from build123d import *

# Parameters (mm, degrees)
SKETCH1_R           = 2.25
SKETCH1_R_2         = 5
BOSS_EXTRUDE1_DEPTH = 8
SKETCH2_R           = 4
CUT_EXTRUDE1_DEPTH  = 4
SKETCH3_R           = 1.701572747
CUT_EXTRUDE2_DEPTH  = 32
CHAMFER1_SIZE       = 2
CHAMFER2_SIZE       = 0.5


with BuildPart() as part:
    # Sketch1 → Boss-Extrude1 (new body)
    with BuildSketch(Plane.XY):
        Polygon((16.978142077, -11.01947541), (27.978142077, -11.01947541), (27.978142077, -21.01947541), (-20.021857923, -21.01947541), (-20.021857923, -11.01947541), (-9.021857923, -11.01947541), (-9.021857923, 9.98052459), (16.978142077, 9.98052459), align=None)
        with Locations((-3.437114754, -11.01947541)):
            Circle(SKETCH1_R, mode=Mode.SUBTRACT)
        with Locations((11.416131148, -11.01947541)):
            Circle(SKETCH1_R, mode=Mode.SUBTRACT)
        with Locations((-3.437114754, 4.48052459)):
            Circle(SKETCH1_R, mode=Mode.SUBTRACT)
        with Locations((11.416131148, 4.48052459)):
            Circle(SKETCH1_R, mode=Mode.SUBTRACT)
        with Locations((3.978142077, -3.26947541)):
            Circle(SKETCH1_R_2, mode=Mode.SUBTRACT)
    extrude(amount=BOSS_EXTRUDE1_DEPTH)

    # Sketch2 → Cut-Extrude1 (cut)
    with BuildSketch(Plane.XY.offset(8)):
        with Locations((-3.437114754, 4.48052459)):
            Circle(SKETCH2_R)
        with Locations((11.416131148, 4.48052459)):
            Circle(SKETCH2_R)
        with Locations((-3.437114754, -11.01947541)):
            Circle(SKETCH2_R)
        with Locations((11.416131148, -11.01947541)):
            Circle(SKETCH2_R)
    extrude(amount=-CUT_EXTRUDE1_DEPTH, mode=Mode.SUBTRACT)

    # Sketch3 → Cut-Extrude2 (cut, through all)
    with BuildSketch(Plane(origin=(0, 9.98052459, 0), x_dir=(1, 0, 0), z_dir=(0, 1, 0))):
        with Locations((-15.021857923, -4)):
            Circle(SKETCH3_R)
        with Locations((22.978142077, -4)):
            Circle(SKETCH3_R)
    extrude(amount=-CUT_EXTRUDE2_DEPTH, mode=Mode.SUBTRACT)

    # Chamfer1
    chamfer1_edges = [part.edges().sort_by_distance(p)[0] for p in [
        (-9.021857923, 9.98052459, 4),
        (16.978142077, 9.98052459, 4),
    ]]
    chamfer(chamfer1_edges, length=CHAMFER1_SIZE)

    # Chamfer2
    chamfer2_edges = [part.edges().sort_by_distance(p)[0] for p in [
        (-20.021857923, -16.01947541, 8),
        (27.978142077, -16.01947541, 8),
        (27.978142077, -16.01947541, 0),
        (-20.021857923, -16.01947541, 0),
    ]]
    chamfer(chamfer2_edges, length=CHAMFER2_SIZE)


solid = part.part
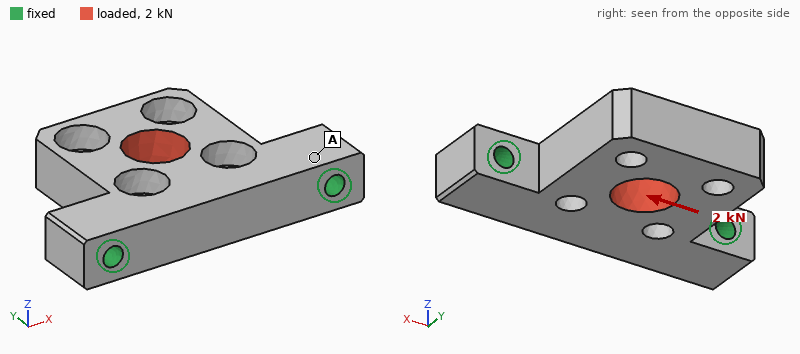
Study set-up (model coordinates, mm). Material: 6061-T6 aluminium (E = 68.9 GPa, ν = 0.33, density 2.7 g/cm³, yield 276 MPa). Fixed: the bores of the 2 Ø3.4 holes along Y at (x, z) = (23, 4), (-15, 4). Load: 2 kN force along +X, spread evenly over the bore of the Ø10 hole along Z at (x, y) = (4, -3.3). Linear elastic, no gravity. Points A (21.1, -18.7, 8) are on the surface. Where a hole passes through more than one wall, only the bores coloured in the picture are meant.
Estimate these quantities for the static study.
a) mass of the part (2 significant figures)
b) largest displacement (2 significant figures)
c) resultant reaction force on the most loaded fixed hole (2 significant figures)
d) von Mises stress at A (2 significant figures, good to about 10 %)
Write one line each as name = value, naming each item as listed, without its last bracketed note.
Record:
mass of the part = 17 g
largest displacement = 22 µm
resultant reaction force on the most loaded fixed hole = 1.3 kN
von Mises stress at A = 9.3 MPa
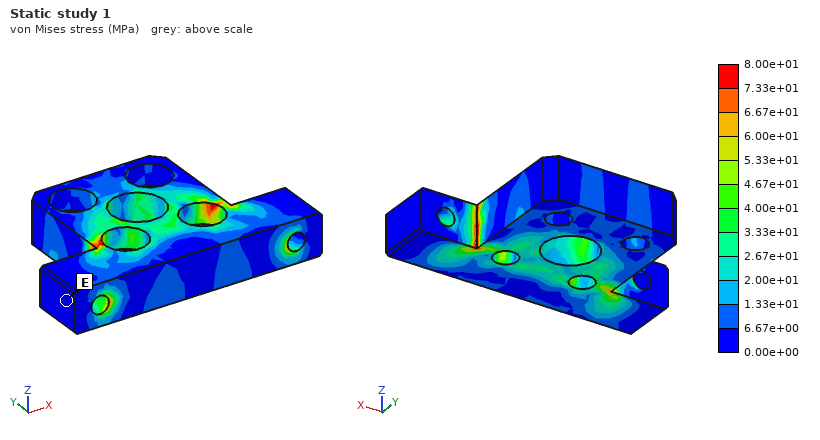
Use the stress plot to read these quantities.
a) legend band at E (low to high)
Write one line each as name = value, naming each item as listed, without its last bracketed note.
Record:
legend band at E = 0.00e+00 to 6.67e+00 MPa
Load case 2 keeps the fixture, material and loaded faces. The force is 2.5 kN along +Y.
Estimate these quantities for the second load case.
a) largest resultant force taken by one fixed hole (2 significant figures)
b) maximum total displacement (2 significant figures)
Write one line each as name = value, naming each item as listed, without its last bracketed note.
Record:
largest resultant force taken by one fixed hole = 1.3 kN
maximum total displacement = 18 µm
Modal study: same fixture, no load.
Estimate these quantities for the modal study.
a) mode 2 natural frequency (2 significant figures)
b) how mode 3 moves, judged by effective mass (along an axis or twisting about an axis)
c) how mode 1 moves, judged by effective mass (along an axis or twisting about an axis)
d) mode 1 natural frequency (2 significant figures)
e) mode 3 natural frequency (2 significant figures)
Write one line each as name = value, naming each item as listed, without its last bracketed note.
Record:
mode 2 natural frequency = 15 kHz
how mode 3 moves, judged by effective mass = along X
how mode 1 moves, judged by effective mass = along Z
mode 1 natural frequency = 5500 Hz
mode 3 natural frequency = 17 kHz
